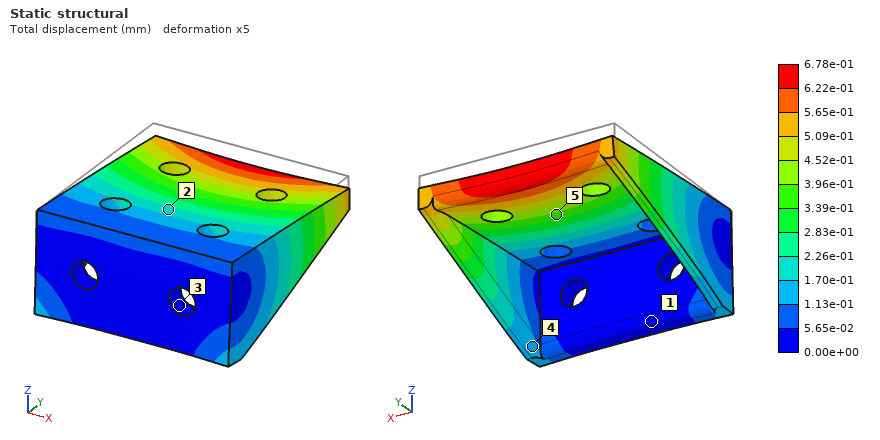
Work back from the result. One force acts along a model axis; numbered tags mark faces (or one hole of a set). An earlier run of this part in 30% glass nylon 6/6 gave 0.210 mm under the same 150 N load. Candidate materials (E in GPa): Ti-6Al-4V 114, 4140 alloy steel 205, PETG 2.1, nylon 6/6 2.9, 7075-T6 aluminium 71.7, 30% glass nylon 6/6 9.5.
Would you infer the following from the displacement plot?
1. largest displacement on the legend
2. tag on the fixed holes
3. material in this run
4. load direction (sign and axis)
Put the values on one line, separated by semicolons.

6.78e-01 mm; 3; nylon 6/6; -Z
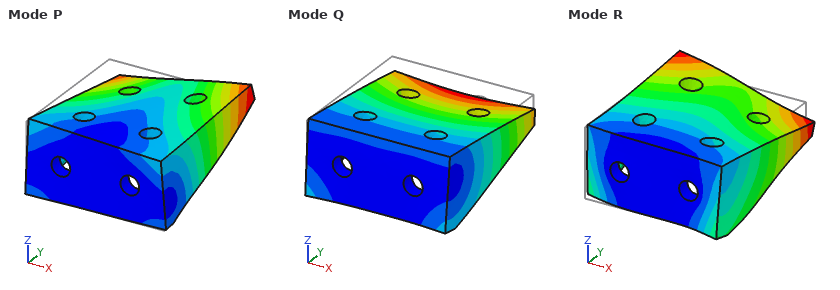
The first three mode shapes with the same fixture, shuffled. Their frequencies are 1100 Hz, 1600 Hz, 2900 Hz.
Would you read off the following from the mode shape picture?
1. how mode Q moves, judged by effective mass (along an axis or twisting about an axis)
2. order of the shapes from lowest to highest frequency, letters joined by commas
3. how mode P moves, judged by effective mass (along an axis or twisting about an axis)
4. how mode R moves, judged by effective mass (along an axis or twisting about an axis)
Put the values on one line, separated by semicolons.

along Z; Q, P, R; along X; along X
